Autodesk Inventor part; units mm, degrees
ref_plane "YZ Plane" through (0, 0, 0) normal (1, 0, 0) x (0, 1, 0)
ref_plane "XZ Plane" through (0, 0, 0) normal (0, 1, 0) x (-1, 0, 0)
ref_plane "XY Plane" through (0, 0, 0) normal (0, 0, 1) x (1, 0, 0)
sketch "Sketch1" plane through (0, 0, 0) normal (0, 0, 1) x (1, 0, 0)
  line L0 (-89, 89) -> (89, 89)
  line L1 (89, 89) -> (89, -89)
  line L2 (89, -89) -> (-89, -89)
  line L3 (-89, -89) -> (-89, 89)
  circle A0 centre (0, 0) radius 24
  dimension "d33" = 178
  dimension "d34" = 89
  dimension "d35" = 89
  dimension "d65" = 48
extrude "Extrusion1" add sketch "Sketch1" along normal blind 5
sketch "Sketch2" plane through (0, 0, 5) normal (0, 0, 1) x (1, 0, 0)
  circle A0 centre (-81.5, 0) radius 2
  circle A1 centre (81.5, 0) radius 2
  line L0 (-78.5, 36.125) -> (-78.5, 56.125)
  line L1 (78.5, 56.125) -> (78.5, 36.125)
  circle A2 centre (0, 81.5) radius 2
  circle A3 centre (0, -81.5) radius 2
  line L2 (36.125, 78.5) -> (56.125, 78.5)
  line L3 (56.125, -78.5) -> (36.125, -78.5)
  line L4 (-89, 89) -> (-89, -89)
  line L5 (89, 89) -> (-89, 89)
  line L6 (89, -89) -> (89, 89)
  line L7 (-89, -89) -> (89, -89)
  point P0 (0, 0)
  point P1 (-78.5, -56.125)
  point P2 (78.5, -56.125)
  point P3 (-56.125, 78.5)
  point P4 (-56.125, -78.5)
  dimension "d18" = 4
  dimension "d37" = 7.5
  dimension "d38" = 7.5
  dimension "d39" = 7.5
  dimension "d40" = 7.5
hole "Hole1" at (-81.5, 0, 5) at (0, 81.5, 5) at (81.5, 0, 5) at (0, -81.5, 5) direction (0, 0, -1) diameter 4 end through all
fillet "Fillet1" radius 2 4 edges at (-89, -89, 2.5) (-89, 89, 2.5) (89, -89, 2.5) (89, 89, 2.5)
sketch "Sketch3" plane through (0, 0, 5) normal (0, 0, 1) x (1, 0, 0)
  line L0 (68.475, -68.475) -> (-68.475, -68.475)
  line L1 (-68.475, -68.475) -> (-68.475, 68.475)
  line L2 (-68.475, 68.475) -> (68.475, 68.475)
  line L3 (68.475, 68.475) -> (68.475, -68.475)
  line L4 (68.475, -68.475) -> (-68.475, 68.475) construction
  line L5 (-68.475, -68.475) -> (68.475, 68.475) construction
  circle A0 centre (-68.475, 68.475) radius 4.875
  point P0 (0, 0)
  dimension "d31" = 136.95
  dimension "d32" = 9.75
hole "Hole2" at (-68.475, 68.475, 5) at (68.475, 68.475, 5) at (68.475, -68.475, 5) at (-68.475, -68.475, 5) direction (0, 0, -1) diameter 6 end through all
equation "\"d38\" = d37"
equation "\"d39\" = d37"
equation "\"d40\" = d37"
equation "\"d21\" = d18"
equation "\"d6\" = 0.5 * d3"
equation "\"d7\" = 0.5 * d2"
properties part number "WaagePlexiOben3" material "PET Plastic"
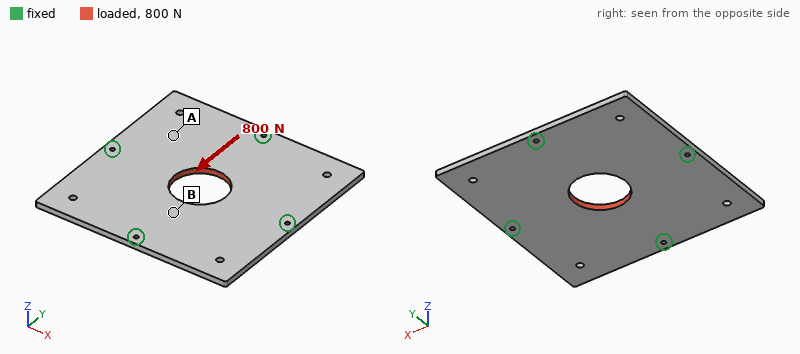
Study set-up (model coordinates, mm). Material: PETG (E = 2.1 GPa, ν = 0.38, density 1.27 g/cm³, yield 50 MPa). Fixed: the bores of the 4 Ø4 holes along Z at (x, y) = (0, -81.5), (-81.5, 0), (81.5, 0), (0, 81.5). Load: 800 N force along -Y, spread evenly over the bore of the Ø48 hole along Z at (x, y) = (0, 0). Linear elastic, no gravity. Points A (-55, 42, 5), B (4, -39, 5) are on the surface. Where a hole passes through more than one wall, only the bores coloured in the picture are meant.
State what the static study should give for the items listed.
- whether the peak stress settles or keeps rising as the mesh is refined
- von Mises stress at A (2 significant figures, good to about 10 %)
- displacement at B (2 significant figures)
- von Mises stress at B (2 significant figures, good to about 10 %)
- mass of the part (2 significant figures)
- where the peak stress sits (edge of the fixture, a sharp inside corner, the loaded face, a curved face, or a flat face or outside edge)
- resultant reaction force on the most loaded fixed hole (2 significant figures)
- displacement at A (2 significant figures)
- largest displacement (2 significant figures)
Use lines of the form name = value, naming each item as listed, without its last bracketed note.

whether the peak stress settles or keeps rising as the mesh is refined = keeps rising
von Mises stress at A = 0.41 MPa
displacement at B = 36 µm
von Mises stress at B = 1.2 MPa
mass of the part = 190 g
where the peak stress sits = edge of the fixture
resultant reaction force on the most loaded fixed hole = 230 N
displacement at A = 26 µm
largest displacement = 49 µm
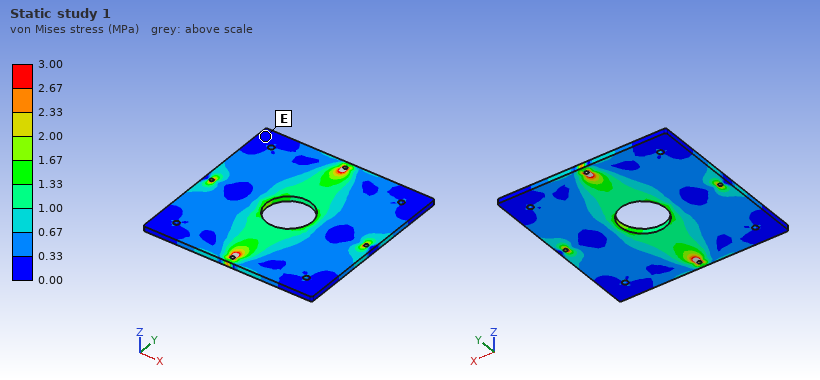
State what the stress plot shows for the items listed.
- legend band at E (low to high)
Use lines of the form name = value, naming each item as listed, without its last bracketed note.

legend band at E = 0.00 to 0.33 MPa
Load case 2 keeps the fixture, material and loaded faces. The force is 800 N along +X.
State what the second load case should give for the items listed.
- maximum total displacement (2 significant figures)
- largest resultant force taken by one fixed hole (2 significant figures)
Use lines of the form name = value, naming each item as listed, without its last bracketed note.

maximum total displacement = 49 µm
largest resultant force taken by one fixed hole = 230 N
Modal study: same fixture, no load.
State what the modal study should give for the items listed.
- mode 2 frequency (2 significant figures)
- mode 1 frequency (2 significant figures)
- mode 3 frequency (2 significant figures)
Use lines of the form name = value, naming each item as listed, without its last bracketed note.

mode 2 frequency = 250 Hz
mode 1 frequency = 220 Hz
mode 3 frequency = 250 Hz
